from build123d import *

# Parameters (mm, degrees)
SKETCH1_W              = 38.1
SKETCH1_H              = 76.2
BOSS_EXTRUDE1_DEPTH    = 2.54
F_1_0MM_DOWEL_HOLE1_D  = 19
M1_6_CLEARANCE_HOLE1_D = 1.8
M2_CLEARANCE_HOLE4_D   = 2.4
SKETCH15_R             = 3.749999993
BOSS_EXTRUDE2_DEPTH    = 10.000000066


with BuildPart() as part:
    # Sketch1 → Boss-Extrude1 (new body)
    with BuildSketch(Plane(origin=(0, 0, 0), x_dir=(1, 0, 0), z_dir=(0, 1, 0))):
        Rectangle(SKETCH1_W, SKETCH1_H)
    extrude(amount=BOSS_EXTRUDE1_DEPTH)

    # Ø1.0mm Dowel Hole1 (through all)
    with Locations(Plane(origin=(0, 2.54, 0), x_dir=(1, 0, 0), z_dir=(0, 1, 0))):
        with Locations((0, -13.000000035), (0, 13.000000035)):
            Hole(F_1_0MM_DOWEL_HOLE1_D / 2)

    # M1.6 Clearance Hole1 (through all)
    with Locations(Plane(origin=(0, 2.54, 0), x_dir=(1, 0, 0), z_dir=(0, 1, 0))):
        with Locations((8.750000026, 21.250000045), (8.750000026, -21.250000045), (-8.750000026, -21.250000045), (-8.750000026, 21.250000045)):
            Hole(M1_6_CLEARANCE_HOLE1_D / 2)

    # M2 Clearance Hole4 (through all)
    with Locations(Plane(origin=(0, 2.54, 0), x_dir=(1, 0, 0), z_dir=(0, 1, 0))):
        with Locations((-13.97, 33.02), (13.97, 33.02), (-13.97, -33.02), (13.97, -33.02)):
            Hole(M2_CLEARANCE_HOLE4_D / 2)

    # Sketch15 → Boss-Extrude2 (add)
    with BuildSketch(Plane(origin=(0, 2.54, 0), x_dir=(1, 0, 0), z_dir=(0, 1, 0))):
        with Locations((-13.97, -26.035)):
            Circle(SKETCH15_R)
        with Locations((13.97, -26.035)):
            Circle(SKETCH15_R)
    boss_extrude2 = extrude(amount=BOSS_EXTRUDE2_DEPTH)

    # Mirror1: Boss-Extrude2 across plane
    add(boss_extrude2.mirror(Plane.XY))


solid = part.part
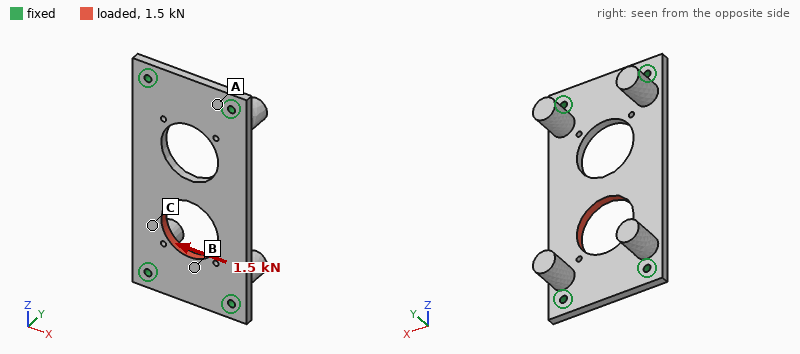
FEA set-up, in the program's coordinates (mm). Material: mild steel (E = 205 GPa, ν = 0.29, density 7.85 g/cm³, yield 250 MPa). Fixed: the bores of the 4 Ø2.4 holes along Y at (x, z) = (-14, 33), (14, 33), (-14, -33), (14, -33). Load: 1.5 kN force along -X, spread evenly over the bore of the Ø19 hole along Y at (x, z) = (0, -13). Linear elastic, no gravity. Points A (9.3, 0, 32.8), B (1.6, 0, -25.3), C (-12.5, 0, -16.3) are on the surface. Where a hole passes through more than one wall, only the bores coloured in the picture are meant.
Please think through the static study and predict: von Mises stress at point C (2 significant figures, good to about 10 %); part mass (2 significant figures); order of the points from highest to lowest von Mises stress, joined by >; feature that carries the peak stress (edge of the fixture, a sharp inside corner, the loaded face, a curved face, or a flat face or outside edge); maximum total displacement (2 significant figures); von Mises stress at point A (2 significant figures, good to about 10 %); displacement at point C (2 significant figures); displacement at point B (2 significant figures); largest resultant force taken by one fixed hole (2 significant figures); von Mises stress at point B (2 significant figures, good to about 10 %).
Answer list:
24 MPa
60 g
B > C > A
edge of the fixture
7.8 µm
9.9 MPa
5.1 µm
2.0 µm
670 N
36 MPa
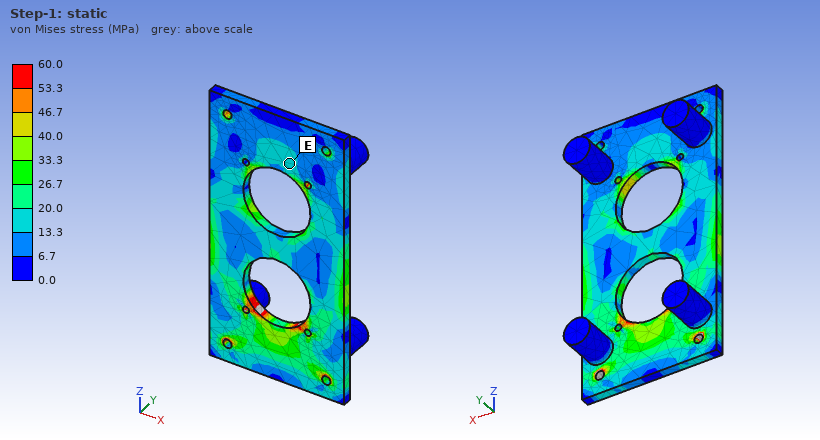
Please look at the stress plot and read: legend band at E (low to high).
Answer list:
13.3 to 20.0 MPa
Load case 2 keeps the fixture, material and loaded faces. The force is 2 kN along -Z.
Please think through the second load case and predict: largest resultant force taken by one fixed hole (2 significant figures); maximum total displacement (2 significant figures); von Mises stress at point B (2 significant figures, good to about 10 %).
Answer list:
710 N
4.0 µm
11 MPa
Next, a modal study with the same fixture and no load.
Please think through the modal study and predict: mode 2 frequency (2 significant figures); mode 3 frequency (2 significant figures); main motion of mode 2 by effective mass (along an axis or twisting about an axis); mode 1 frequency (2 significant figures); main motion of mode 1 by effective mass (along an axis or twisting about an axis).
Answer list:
4200 Hz
6800 Hz
twisting about Z
3000 Hz
along Y
